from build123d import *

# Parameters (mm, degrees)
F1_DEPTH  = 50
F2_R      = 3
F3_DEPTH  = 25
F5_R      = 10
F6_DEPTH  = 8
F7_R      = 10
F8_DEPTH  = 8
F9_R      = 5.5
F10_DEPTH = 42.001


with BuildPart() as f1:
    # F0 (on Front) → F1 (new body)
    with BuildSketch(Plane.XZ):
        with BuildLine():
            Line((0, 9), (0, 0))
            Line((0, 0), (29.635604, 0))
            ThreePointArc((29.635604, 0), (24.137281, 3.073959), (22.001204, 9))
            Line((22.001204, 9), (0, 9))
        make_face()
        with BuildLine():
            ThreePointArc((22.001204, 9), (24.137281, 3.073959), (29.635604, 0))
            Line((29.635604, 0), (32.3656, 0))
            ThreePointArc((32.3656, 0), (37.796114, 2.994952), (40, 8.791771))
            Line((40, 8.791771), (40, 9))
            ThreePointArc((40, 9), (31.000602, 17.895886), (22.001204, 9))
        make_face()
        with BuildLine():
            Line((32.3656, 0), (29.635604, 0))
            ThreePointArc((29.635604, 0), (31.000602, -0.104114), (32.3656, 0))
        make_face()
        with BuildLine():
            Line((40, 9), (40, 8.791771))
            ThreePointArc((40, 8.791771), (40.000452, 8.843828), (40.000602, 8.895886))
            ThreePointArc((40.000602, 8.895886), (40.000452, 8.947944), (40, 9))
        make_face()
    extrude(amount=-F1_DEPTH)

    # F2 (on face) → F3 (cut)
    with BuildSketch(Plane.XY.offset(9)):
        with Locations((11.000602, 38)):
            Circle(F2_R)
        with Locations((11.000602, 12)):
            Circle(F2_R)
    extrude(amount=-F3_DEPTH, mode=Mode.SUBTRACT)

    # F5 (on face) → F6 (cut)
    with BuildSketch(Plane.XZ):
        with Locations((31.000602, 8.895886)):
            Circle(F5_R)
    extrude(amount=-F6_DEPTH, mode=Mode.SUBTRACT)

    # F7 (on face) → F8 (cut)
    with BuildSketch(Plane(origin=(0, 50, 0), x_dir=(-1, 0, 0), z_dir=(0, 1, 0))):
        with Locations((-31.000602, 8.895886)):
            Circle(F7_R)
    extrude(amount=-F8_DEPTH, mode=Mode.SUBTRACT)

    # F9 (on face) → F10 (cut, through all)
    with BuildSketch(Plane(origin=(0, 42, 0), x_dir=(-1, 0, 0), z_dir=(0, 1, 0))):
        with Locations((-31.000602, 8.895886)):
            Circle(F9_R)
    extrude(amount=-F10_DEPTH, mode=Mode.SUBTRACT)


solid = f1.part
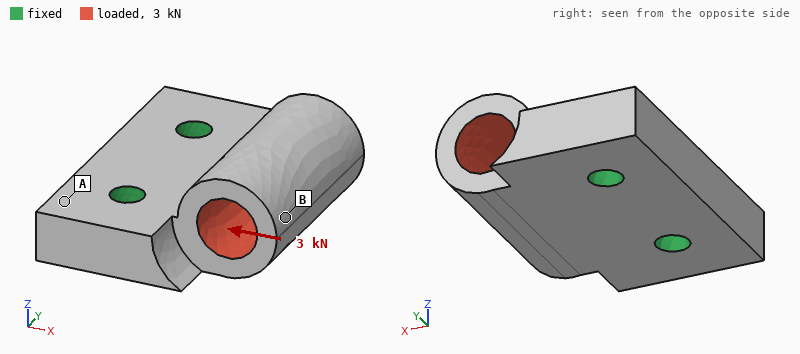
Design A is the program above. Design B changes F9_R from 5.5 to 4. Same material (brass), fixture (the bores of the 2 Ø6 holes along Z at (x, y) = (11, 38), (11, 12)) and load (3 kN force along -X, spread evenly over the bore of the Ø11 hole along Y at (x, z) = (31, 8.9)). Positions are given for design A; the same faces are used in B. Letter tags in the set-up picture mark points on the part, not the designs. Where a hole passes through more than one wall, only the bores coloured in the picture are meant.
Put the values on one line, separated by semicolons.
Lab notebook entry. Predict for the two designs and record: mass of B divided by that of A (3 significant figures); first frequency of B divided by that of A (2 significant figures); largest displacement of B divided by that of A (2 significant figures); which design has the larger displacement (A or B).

1.10; 0.99; 0.72; A
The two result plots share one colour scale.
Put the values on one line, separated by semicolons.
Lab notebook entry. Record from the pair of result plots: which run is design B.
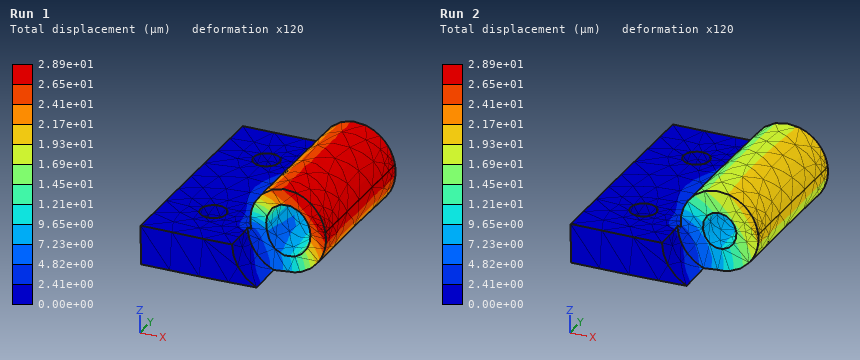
Run 2
